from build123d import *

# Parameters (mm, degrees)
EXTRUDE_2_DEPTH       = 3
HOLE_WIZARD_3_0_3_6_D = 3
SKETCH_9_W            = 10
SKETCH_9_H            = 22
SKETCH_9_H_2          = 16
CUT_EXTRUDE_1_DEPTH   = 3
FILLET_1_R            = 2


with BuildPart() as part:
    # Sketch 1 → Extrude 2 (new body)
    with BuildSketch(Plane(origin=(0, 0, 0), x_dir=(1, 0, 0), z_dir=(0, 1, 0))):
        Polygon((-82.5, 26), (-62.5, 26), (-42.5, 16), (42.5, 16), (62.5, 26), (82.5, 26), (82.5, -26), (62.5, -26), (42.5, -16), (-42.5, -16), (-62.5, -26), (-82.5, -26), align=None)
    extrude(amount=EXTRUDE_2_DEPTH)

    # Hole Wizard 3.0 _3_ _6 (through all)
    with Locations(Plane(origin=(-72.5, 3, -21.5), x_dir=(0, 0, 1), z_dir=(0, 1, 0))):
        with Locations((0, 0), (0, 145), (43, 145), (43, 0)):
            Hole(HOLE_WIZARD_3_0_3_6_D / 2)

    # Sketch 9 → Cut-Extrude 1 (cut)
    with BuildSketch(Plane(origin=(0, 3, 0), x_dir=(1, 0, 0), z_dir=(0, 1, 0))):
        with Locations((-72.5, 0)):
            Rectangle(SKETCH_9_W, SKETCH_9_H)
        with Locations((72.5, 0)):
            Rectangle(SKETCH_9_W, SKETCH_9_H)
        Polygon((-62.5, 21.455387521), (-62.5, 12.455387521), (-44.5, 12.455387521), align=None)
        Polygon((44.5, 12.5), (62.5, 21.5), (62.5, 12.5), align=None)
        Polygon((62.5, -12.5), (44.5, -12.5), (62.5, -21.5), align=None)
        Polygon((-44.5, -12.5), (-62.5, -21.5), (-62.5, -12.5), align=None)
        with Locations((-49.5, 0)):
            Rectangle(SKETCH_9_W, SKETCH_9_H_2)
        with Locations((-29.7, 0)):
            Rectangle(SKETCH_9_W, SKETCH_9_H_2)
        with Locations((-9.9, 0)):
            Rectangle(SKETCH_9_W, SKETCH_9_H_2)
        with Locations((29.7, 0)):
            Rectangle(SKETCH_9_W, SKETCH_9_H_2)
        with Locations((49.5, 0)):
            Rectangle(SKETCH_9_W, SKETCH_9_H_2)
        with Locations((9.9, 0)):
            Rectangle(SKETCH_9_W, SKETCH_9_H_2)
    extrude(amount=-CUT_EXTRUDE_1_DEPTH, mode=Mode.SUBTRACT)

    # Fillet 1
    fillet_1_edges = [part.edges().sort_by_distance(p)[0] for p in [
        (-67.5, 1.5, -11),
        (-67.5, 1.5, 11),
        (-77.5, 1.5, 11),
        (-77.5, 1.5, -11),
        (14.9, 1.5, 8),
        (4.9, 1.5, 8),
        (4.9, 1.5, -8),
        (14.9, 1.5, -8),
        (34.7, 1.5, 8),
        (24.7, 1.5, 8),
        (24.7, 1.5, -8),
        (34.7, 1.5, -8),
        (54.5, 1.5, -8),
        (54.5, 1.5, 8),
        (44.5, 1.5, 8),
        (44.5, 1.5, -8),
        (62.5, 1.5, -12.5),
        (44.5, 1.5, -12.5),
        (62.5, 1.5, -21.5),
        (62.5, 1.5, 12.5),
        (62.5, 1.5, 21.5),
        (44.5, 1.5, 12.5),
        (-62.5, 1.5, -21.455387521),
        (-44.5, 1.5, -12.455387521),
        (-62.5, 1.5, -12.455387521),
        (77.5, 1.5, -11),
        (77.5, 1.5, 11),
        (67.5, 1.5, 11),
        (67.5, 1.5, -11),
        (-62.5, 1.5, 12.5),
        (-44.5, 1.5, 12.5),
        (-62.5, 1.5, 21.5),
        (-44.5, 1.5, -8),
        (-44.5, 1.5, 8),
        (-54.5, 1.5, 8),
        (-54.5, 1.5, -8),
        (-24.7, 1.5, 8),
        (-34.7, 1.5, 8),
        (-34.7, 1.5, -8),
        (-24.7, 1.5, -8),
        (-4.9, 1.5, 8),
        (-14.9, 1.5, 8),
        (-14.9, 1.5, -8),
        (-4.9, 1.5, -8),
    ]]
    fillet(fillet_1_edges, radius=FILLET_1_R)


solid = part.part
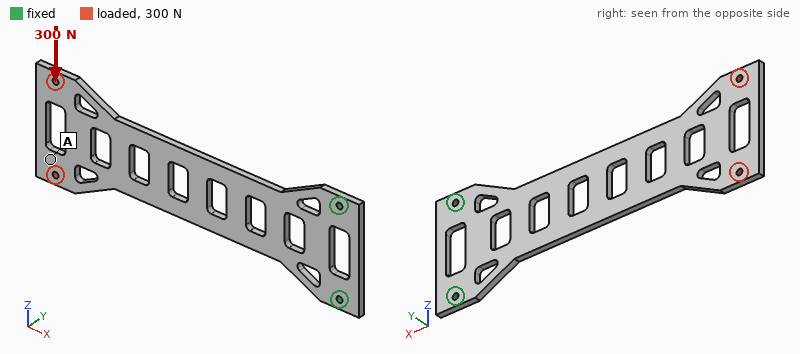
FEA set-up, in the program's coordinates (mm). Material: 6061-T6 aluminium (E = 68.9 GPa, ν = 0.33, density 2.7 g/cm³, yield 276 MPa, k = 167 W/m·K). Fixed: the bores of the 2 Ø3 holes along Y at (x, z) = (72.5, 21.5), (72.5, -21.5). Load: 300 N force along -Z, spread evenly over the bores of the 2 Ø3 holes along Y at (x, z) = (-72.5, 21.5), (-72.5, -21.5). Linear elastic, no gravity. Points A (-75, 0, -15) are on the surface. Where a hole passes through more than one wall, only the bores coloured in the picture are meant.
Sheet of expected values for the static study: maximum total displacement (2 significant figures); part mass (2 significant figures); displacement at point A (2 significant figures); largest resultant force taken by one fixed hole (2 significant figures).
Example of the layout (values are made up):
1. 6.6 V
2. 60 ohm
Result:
1. 0.65 mm
2. 39 g
3. 0.60 mm
4. 1.0 kN
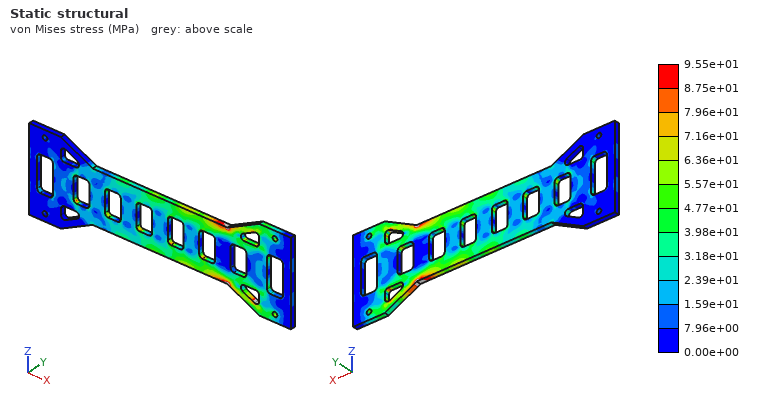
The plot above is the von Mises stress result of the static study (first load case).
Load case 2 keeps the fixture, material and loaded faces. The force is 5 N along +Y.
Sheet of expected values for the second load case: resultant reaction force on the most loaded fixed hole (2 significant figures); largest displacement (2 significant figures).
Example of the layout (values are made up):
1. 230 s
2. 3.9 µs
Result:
1. 2.5 N
2. 1.8 mm
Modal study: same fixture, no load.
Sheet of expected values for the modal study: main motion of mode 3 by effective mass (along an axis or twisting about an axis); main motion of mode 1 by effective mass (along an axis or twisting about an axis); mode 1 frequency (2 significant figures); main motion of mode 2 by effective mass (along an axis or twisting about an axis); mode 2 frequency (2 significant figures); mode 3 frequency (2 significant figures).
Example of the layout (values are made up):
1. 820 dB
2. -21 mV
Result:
1. twisting about X
2. along Y
3. 80 Hz
4. along Y
5. 540 Hz
6. 580 Hz
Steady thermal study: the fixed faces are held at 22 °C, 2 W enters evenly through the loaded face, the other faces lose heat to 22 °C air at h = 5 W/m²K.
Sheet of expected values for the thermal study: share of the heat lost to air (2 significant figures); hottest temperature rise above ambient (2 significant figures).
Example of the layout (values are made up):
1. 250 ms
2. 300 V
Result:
1. 34 %
2. 23 K
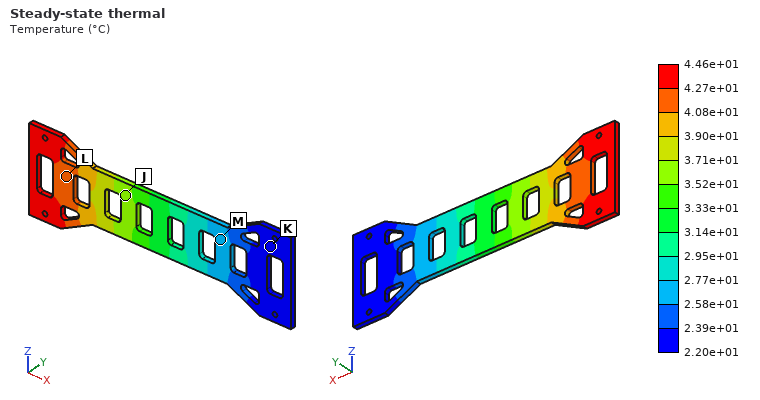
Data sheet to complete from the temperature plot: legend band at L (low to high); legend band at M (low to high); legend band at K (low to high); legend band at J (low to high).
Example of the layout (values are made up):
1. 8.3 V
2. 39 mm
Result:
1. 4.08e+01 to 4.27e+01 °C
2. 2.58e+01 to 2.77e+01 °C
3. 2.20e+01 to 2.39e+01 °C
4. 3.52e+01 to 3.71e+01 °C
